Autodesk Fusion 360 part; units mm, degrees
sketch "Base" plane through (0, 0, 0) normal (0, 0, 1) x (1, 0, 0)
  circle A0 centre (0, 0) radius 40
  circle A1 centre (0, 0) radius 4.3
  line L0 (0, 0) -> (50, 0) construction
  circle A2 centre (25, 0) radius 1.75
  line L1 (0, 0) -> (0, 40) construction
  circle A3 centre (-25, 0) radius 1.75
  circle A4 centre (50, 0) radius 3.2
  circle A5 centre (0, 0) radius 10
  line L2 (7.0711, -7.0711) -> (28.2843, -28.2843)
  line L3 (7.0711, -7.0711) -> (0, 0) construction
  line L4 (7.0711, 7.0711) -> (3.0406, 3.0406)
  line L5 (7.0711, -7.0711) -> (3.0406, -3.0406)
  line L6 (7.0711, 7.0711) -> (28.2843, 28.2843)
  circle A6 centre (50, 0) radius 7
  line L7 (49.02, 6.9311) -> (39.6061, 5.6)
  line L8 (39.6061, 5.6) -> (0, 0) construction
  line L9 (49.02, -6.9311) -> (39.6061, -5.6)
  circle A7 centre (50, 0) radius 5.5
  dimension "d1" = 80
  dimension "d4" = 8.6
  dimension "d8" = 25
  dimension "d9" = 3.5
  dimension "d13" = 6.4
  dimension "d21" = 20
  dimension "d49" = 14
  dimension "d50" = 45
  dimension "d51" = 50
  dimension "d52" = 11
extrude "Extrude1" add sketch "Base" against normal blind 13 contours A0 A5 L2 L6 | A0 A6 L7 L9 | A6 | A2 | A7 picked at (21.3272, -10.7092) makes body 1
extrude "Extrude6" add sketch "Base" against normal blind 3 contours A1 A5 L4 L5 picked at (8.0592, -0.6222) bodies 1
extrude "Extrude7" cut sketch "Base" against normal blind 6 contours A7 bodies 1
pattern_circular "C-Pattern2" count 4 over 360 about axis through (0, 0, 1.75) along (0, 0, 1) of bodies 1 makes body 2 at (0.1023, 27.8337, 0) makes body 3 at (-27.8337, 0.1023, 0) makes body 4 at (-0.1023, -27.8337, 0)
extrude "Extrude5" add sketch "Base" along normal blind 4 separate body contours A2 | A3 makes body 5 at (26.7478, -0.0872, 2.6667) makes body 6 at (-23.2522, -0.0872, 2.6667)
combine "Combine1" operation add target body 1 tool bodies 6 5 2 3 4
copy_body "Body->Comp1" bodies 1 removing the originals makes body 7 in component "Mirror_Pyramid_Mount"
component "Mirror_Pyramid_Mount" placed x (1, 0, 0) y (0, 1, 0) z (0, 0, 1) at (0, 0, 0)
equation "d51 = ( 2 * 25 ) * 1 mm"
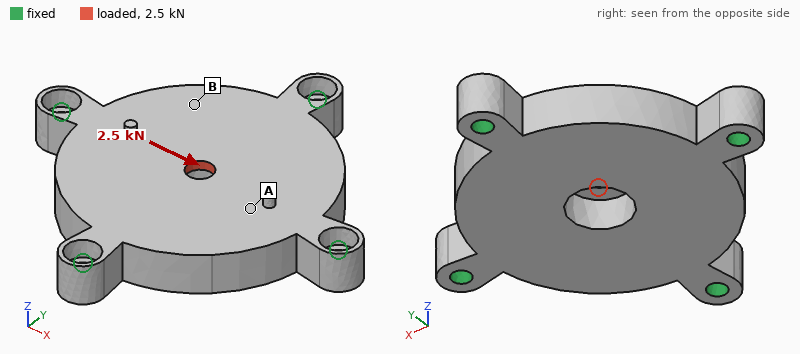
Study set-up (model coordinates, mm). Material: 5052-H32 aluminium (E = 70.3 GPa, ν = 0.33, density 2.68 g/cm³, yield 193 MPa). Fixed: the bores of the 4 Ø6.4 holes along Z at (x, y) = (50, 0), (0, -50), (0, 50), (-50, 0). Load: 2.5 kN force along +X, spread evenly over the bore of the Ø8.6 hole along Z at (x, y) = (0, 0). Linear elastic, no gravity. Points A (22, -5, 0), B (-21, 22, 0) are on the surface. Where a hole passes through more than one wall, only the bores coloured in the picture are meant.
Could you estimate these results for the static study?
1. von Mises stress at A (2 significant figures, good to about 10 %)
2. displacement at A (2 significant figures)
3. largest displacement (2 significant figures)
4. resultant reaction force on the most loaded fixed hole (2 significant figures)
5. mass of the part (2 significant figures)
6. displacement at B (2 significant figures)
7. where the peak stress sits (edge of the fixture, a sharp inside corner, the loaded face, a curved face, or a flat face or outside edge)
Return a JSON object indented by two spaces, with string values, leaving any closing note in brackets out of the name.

{
  "von Mises stress at A": "6.4 MPa",
  "displacement at A": "2.6 µm",
  "largest displacement": "7.0 µm",
  "resultant reaction force on the most loaded fixed hole": "1.0 kN",
  "mass of the part": "190 g",
  "displacement at B": "2.7 µm",
  "where the peak stress sits": "the loaded face"
}
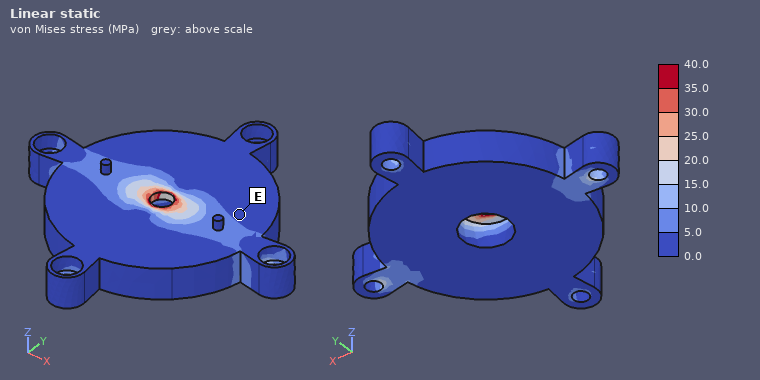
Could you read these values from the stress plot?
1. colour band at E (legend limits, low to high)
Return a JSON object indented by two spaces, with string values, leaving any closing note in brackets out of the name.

{
  "colour band at E": "0.0 to 5.0 MPa"
}
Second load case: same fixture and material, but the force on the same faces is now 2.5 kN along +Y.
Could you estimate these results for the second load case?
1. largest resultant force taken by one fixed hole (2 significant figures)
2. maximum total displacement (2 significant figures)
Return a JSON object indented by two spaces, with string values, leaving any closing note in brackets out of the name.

{
  "largest resultant force taken by one fixed hole": "1.0 kN",
  "maximum total displacement": "7.0 µm"
}
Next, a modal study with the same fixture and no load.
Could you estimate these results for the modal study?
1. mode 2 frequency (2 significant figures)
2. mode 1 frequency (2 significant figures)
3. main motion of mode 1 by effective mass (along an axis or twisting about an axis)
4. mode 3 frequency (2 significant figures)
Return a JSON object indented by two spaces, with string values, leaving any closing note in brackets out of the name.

{
  "mode 2 frequency": "9200 Hz",
  "mode 1 frequency": "6000 Hz",
  "main motion of mode 1 by effective mass": "along Z",
  "mode 3 frequency": "9200 Hz"
}
